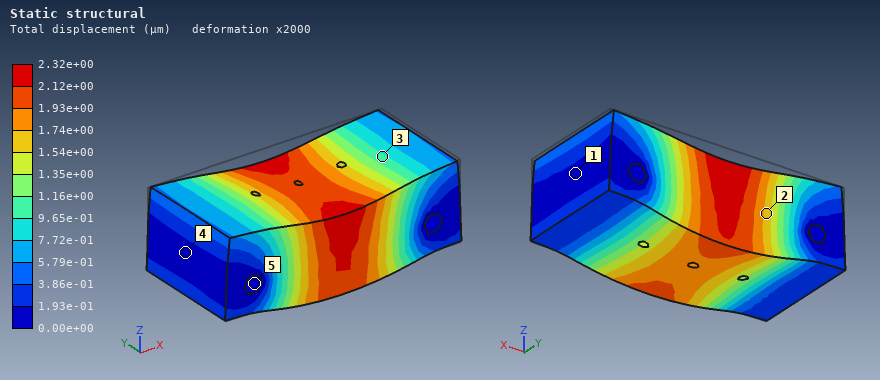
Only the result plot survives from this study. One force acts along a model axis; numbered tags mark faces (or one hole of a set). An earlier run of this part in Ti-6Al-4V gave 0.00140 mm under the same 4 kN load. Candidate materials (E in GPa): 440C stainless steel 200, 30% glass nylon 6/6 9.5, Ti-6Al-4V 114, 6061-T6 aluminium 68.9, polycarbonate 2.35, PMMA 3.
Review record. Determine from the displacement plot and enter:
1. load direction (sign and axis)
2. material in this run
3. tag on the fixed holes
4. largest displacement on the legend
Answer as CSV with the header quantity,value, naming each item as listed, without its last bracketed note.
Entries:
quantity,value
load direction,-Z
material in this run,6061-T6 aluminium
tag on the fixed holes,5
largest displacement on the legend,2.32e+00 µm
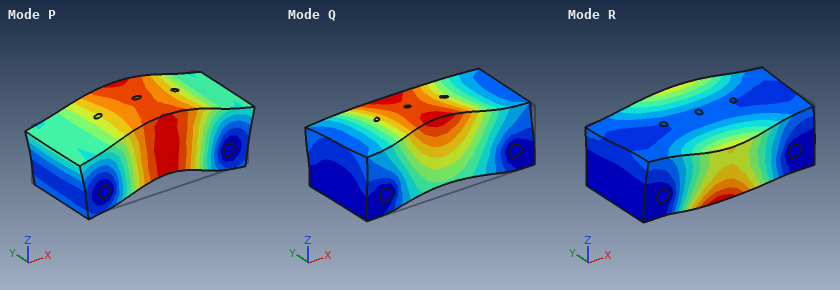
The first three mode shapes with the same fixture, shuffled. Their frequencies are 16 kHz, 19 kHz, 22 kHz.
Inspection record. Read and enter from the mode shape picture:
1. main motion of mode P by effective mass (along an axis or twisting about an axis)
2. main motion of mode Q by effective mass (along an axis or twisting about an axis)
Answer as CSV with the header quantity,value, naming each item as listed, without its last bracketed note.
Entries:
quantity,value
main motion of mode P by effective mass,along Z
main motion of mode Q by effective mass,along Y
